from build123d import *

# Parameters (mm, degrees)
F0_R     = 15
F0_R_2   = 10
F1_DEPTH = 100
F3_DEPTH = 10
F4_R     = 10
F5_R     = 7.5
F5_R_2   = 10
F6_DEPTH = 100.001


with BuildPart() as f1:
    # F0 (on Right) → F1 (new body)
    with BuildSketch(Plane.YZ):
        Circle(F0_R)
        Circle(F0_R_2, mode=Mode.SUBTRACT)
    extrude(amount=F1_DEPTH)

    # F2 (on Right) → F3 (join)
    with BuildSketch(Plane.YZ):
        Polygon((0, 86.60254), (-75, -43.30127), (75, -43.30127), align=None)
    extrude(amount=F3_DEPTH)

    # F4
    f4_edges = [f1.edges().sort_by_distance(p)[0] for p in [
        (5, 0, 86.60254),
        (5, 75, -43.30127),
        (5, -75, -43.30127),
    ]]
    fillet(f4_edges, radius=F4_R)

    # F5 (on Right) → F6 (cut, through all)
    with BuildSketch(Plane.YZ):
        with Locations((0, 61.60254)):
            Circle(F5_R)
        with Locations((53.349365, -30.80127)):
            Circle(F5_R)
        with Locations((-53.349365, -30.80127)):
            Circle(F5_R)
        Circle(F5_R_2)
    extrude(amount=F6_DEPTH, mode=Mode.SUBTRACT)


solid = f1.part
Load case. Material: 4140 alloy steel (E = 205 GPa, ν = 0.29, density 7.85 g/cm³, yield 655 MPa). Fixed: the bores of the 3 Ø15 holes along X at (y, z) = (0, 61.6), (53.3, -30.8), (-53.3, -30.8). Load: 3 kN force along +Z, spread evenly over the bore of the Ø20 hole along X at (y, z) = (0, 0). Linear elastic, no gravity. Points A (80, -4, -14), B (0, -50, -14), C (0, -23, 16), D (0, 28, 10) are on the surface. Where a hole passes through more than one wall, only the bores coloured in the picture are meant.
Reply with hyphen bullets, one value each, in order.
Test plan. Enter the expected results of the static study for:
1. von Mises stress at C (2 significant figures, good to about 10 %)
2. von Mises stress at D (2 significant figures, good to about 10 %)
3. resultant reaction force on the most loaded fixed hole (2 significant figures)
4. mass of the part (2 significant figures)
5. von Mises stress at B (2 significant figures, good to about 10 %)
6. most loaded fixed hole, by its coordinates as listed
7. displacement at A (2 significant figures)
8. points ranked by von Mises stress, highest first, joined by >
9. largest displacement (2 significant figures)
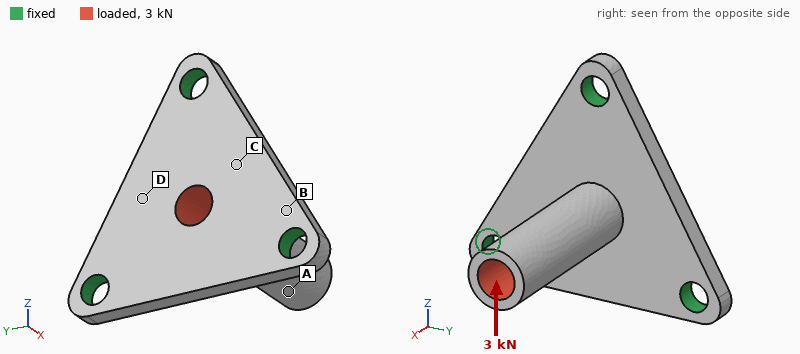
- 27 MPa
- 21 MPa
- 2.3 kN
- 960 g
- 12 MPa
- (0, 61.6)
- 0.10 mm
- C > D > B > A
- 0.13 mm
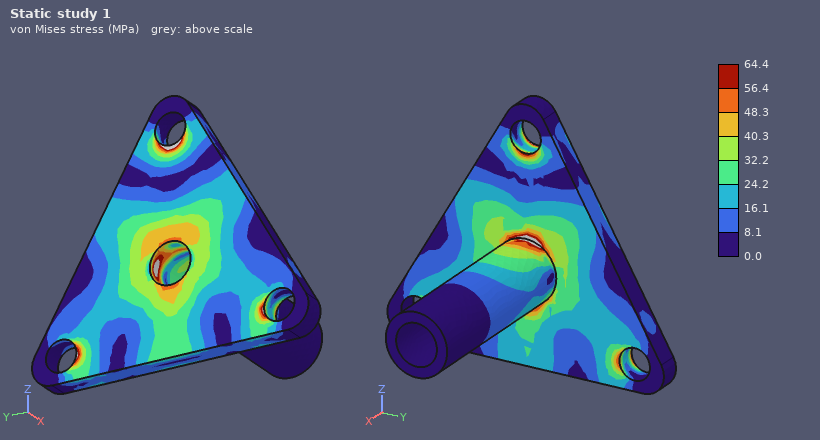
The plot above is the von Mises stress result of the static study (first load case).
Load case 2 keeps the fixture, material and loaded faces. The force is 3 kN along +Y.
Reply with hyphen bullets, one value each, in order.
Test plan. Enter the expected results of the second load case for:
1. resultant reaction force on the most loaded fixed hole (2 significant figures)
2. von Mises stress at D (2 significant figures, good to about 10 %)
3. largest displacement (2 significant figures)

- 2.0 kN
- 29 MPa
- 0.13 mm
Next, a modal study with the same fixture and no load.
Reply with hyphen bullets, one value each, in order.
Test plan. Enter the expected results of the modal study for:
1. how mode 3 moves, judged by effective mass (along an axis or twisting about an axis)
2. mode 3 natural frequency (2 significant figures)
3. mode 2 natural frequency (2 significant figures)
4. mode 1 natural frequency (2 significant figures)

- along X
- 3200 Hz
- 1700 Hz
- 1700 Hz
